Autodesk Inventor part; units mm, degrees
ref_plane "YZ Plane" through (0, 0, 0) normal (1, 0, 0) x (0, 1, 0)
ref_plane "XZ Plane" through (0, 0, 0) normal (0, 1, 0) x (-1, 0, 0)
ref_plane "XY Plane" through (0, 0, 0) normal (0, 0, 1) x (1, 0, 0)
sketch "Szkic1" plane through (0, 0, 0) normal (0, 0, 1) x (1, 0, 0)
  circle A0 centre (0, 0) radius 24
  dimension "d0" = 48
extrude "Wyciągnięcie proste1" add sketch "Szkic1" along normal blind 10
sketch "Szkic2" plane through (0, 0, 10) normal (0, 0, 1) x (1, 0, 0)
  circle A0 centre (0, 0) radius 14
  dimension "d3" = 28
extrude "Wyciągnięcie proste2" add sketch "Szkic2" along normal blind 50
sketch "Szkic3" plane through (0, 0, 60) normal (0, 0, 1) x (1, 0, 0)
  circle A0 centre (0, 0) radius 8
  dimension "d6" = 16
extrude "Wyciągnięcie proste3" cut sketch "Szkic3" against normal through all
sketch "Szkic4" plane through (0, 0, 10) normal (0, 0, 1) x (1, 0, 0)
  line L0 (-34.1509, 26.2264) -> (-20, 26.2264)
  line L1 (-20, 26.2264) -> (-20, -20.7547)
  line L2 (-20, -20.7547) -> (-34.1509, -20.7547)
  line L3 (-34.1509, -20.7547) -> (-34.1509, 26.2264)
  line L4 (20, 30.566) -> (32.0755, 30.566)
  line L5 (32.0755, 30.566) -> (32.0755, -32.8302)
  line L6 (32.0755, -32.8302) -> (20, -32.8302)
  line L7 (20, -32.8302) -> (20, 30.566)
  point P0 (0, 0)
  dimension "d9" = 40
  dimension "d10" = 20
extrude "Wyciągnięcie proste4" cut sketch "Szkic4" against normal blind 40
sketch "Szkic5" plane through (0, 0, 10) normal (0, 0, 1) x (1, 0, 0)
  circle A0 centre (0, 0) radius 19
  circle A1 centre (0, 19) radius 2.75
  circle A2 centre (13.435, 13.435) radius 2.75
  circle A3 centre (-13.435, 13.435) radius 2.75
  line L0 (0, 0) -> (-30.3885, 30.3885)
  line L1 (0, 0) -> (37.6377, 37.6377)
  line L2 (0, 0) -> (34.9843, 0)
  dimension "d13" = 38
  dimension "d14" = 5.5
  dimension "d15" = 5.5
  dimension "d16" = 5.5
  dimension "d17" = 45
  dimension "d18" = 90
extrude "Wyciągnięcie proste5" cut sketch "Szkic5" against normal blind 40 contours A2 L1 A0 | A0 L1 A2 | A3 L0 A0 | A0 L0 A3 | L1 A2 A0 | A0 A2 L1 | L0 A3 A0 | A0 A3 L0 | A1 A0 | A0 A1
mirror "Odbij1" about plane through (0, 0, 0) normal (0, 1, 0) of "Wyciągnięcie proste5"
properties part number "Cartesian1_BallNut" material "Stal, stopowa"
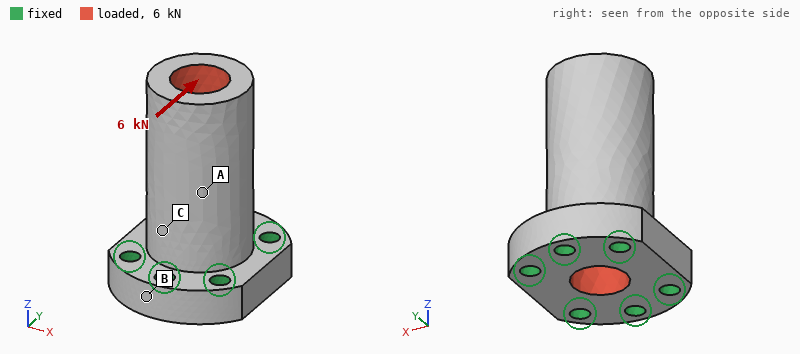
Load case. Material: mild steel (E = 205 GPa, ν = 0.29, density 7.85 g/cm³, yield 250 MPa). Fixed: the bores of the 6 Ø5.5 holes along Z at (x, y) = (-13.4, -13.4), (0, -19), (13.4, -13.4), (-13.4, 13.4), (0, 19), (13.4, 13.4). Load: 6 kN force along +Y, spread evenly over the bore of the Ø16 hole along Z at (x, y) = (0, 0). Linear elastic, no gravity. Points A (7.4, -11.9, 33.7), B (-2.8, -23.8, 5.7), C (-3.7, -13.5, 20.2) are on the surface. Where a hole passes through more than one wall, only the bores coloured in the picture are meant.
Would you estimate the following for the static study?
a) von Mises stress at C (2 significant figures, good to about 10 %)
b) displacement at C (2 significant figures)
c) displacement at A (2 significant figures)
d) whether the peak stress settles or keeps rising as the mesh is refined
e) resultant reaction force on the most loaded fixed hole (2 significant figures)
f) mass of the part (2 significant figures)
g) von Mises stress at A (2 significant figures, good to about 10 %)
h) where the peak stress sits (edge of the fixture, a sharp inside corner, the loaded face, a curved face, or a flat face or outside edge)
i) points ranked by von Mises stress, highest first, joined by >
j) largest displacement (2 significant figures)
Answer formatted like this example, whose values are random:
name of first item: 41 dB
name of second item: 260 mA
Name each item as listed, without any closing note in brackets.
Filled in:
von Mises stress at C: 37 MPa
displacement at C: 7.3 µm
displacement at A: 14 µm
whether the peak stress settles or keeps rising as the mesh is refined: keeps rising
resultant reaction force on the most loaded fixed hole: 2.6 kN
mass of the part: 270 g
von Mises stress at A: 17 MPa
where the peak stress sits: a sharp inside corner
points ranked by von Mises stress, highest first, joined by >: C > A > B
largest displacement: 29 µm
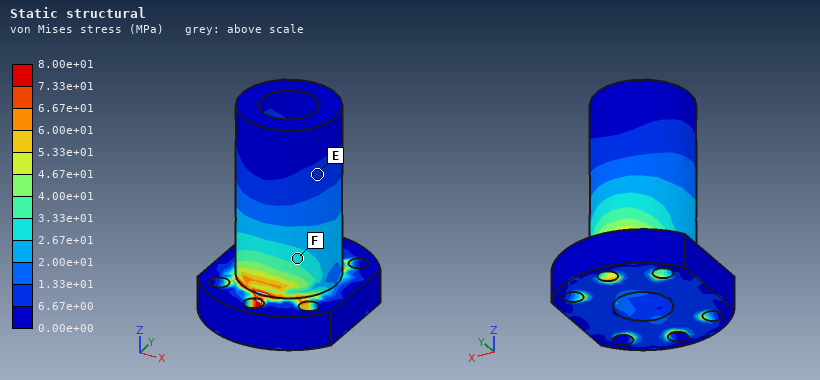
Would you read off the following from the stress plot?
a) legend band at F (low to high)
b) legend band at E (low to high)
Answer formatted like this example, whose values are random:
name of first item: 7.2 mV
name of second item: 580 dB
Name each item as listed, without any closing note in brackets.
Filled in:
legend band at F: 2.67e+01 to 3.33e+01 MPa
legend band at E: 6.67e+00 to 1.33e+01 MPa
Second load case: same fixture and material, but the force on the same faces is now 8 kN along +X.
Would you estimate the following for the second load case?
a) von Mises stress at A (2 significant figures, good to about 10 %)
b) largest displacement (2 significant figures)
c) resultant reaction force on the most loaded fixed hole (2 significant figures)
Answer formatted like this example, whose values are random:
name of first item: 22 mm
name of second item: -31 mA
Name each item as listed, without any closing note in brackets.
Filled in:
von Mises stress at A: 23 MPa
largest displacement: 44 µm
resultant reaction force on the most loaded fixed hole: 4.2 kN
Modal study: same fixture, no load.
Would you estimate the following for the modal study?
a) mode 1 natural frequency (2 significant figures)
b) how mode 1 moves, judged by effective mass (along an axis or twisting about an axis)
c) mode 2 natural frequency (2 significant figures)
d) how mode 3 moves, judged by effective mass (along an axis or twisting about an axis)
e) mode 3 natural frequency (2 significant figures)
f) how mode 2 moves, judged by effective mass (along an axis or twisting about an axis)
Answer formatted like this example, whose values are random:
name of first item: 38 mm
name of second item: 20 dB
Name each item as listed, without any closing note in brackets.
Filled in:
mode 1 natural frequency: 5800 Hz
how mode 1 moves, judged by effective mass: along X
mode 2 natural frequency: 6200 Hz
how mode 3 moves, judged by effective mass: twisting about Z
mode 3 natural frequency: 15 kHz
how mode 2 moves, judged by effective mass: along Y
